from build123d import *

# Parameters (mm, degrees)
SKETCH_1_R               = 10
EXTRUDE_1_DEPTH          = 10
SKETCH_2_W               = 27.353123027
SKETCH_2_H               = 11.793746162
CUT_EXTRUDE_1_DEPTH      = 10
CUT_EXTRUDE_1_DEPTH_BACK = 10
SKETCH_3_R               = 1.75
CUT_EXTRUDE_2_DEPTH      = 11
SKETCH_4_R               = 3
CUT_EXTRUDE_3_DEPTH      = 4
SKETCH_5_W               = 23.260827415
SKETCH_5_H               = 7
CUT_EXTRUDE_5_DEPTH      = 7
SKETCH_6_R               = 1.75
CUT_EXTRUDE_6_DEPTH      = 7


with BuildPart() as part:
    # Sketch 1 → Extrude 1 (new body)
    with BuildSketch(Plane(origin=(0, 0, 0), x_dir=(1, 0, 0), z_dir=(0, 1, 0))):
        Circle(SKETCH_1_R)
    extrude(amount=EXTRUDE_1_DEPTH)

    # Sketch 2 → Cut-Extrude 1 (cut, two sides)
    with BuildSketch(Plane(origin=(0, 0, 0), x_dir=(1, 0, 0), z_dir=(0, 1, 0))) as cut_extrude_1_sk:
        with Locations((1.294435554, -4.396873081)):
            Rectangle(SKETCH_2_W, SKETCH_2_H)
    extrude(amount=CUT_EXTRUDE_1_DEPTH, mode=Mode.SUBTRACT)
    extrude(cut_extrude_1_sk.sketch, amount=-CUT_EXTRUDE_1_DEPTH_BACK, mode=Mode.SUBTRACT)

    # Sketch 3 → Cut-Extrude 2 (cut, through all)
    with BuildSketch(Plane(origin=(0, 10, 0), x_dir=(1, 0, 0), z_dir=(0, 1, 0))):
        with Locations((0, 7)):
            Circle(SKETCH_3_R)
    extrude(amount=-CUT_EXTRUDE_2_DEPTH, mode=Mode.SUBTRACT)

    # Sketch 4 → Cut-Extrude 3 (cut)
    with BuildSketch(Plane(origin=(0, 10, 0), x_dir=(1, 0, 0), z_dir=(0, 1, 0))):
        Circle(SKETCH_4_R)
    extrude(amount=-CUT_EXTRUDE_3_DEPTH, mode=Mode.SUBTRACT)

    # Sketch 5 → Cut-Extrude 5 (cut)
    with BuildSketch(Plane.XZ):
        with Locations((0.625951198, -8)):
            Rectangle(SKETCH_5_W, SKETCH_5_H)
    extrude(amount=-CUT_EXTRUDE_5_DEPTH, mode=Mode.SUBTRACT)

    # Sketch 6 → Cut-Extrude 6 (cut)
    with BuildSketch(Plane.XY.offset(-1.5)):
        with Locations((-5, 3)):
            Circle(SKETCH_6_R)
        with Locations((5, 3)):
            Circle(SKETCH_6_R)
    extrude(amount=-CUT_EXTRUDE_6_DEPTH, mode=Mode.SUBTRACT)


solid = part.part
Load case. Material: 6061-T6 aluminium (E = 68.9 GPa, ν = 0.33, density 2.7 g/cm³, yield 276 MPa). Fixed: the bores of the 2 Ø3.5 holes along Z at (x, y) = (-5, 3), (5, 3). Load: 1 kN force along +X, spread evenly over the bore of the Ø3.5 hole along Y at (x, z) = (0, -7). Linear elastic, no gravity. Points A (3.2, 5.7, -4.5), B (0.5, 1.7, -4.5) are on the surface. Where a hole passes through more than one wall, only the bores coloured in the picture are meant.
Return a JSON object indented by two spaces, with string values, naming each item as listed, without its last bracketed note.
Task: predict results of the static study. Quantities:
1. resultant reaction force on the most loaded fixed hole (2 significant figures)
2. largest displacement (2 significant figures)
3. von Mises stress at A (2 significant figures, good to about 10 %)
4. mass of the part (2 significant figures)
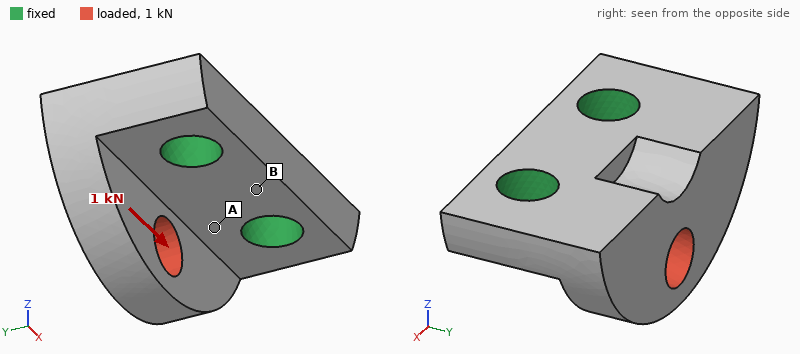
{
  "resultant reaction force on the most loaded fixed hole": "680 N",
  "largest displacement": "18 µm",
  "von Mises stress at A": "79 MPa",
  "mass of the part": "1.8 g"
}
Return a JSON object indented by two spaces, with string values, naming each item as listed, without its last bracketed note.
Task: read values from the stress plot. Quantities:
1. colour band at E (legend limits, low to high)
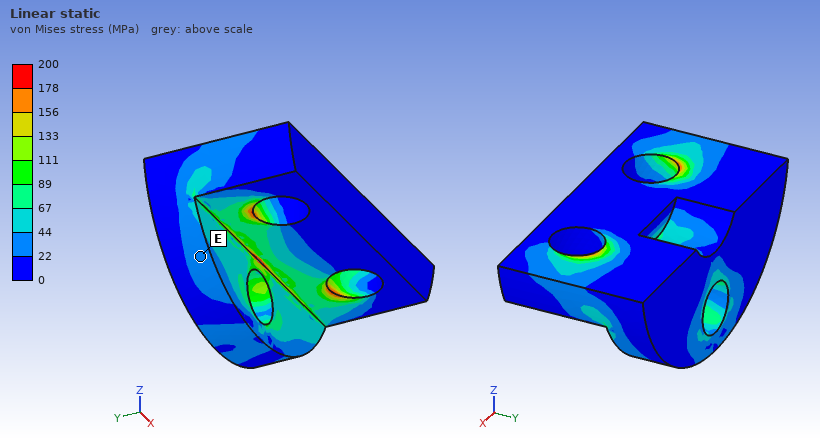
{
  "colour band at E": "22 to 44 MPa"
}
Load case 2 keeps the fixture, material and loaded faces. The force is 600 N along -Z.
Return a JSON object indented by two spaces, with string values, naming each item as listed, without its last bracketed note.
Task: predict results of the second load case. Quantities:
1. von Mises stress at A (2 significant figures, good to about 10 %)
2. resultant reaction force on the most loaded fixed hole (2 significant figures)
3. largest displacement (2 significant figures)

{
  "von Mises stress at A": "65 MPa",
  "resultant reaction force on the most loaded fixed hole": "300 N",
  "largest displacement": "25 µm"
}
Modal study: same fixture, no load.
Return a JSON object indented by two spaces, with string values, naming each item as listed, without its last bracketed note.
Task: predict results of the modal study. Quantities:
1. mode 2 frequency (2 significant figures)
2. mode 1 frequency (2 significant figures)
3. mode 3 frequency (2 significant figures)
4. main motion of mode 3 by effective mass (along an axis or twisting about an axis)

{
  "mode 2 frequency": "45 kHz",
  "mode 1 frequency": "30 kHz",
  "mode 3 frequency": "66 kHz",
  "main motion of mode 3 by effective mass": "along X"
}
